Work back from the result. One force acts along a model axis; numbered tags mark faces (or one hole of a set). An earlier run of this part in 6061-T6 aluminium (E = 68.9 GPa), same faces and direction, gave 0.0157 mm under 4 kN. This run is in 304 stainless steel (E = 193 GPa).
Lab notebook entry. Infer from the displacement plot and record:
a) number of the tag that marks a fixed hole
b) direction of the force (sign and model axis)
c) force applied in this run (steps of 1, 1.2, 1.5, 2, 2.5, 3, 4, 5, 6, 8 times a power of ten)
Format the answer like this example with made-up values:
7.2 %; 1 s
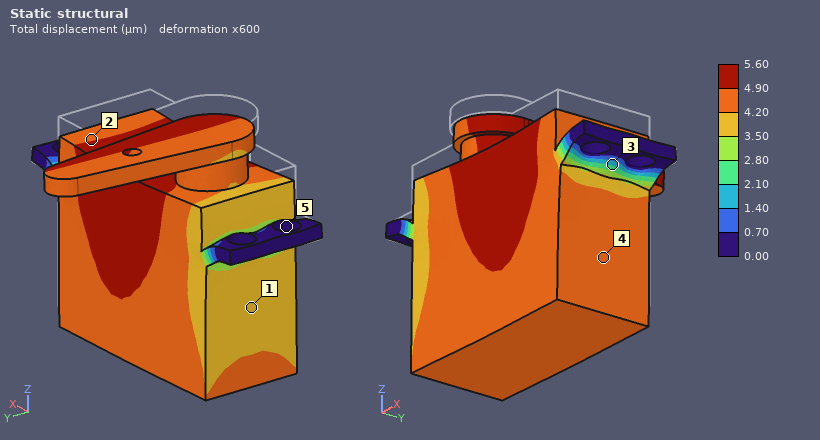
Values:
5; -Z; 4 kN
